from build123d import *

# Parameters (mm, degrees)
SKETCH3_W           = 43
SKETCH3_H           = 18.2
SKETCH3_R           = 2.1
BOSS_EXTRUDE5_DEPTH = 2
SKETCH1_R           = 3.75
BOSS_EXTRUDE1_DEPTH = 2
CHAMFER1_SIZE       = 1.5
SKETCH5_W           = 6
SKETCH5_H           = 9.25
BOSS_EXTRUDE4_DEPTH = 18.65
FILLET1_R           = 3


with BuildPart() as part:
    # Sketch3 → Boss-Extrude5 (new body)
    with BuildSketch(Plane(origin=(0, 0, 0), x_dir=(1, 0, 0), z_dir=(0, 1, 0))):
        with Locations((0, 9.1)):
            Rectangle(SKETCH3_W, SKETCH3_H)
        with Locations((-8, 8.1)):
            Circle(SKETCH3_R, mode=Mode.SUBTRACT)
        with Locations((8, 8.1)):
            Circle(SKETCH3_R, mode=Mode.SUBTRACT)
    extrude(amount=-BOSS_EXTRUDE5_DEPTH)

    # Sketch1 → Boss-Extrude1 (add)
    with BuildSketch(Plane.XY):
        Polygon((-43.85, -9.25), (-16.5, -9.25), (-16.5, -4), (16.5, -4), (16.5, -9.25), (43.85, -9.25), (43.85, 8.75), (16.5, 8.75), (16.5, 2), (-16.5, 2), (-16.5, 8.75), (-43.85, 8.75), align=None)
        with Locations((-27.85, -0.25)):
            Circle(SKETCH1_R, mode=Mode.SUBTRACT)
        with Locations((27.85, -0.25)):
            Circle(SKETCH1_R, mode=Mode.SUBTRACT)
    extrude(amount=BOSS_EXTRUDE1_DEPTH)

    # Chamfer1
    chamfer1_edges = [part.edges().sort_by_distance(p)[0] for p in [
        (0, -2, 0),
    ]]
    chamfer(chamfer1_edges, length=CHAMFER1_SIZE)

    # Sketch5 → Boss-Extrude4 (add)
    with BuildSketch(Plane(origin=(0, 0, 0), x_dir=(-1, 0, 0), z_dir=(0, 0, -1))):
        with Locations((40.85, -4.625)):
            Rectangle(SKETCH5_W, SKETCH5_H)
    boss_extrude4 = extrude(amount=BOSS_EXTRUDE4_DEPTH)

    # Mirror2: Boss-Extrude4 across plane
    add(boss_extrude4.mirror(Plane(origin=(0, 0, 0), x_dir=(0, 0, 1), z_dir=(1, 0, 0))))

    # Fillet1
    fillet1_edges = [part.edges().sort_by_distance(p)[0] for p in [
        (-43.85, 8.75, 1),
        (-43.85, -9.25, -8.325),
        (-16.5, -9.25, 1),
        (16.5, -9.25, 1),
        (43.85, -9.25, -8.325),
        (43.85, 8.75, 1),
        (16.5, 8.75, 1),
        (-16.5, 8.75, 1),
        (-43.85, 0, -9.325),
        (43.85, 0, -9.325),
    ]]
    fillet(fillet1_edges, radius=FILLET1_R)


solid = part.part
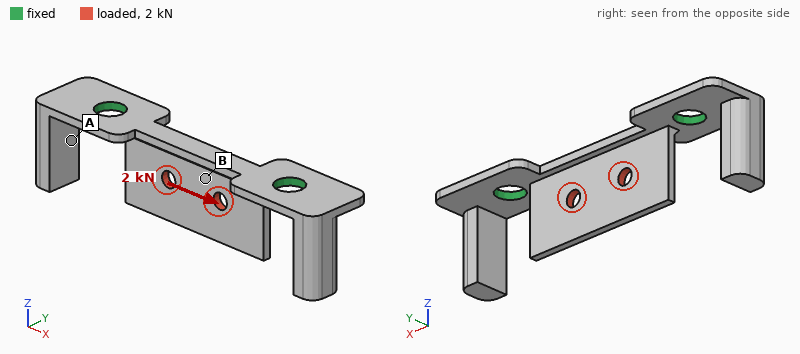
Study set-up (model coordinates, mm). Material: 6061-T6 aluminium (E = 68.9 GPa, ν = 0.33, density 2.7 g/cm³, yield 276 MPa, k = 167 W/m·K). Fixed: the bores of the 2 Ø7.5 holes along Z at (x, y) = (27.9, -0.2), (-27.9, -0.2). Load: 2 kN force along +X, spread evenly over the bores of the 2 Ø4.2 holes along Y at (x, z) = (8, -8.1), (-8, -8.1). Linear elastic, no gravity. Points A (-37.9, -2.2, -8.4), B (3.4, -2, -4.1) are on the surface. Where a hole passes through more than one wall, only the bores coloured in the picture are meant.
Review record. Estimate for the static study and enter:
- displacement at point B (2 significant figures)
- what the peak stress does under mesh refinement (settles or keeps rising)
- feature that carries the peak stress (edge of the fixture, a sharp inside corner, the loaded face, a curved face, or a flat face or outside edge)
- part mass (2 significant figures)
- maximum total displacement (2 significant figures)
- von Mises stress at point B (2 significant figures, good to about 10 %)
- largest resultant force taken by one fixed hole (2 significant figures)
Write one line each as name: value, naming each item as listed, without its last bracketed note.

displacement at point B: 15 µm
what the peak stress does under mesh refinement: keeps rising
feature that carries the peak stress: edge of the fixture
part mass: 15 g
maximum total displacement: 31 µm
von Mises stress at point B: 40 MPa
largest resultant force taken by one fixed hole: 1.1 kN
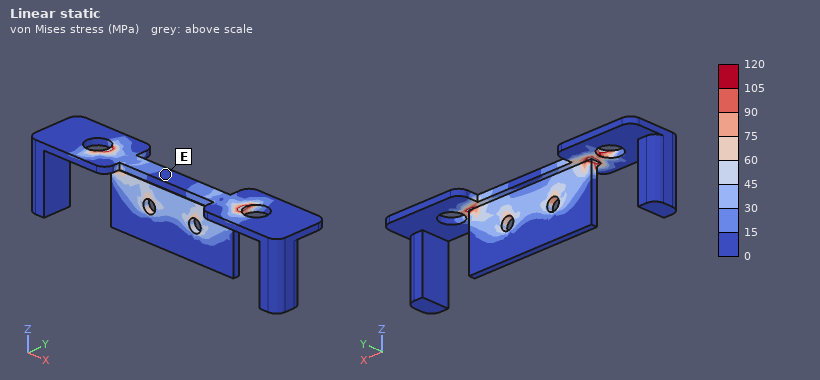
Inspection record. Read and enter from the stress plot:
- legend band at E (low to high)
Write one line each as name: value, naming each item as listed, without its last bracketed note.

legend band at E: 0 to 15 MPa
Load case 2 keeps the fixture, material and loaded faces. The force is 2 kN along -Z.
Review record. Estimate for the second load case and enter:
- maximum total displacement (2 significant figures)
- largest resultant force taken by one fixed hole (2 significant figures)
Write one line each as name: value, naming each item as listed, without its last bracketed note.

maximum total displacement: 70 µm
largest resultant force taken by one fixed hole: 1.3 kN
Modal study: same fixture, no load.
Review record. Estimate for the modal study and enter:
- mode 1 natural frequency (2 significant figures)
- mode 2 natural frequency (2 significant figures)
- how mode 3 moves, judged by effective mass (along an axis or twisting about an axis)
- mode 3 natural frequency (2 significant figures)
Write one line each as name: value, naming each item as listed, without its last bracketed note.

mode 1 natural frequency: 2200 Hz
mode 2 natural frequency: 2200 Hz
how mode 3 moves, judged by effective mass: along Y
mode 3 natural frequency: 2800 Hz
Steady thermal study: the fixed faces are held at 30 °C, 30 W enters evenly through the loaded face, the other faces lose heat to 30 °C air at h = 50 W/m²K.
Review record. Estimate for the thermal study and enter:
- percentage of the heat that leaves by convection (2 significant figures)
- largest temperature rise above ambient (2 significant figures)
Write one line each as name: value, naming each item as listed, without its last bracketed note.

percentage of the heat that leaves by convection: 16 %
largest temperature rise above ambient: 58 K
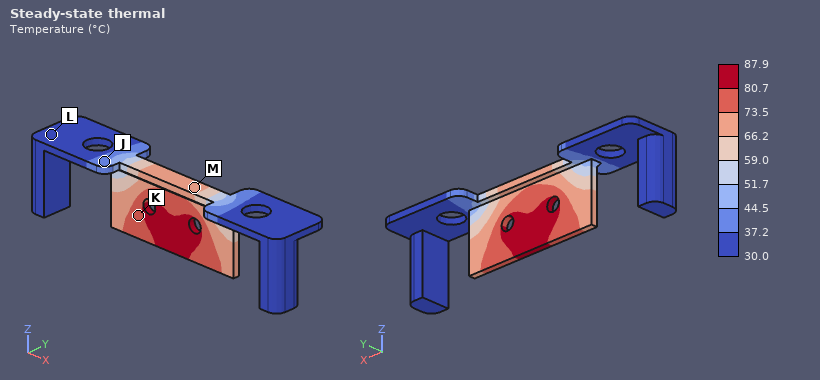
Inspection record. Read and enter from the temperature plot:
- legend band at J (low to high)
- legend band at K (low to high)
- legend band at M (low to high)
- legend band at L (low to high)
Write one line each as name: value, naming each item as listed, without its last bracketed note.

legend band at J: 37.2 to 44.5 °C
legend band at K: 73.5 to 80.7 °C
legend band at M: 66.2 to 73.5 °C
legend band at L: 30.0 to 37.2 °C
